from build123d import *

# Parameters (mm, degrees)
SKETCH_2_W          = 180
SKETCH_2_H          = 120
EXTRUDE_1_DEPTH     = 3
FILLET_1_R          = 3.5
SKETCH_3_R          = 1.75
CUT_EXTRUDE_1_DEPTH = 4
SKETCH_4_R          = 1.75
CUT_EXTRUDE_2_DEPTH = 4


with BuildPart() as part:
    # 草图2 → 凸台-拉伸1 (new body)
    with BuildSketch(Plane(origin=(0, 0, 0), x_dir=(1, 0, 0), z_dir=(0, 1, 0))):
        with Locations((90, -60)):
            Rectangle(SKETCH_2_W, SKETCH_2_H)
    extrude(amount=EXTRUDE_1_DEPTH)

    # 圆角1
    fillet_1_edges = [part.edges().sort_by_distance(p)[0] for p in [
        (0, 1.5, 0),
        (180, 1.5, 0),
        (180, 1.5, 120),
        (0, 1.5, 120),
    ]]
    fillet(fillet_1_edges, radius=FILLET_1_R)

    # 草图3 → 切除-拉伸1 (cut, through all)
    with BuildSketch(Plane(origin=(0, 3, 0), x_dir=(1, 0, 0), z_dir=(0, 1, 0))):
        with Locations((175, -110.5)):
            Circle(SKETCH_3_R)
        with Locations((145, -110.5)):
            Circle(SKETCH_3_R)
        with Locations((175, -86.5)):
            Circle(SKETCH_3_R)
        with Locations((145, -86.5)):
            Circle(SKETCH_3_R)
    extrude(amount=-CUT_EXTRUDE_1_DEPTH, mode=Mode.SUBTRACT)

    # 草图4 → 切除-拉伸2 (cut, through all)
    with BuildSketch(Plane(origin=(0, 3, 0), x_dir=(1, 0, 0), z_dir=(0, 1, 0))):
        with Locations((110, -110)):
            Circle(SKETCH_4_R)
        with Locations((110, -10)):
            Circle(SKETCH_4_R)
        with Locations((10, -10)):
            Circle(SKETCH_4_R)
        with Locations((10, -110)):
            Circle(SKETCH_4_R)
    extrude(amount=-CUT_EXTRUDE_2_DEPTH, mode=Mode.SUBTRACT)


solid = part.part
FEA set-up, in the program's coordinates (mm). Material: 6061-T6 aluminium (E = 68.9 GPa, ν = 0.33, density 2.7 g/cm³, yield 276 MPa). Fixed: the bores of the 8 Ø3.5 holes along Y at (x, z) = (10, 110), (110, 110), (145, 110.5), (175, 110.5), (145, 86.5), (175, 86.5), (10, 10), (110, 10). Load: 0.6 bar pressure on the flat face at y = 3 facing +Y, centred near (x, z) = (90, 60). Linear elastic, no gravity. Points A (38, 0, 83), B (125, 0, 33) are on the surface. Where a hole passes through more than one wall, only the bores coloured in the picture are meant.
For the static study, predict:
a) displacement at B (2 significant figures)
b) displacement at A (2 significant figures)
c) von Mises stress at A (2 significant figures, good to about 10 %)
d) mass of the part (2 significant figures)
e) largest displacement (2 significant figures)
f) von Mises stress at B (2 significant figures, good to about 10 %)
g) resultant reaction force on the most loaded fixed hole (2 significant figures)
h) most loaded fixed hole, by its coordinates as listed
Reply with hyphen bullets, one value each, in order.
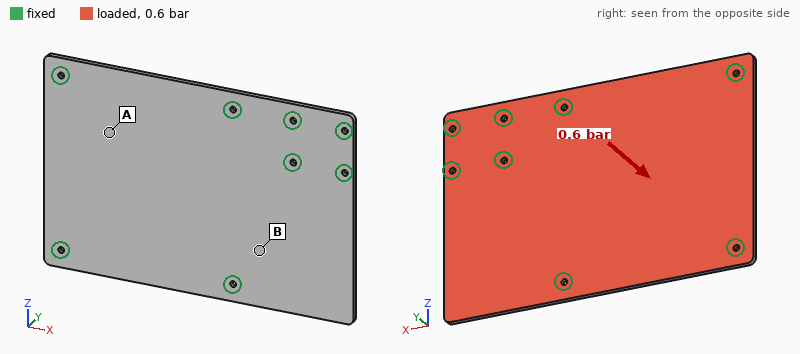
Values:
- 0.096 mm
- 0.20 mm
- 16 MPa
- 170 g
- 0.49 mm
- 30 MPa
- 350 N
- (110, 10)
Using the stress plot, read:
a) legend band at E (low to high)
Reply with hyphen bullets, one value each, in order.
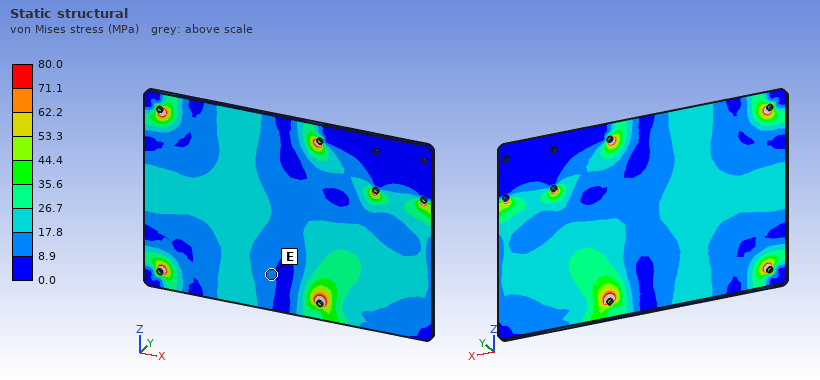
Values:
- 8.9 to 17.8 MPa
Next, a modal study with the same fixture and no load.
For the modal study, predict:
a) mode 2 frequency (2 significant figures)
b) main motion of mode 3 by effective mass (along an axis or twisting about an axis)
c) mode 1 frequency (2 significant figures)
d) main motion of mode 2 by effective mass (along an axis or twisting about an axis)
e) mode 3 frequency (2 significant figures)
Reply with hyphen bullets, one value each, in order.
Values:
- 1000 Hz
- twisting about X
- 800 Hz
- along Y
- 1700 Hz
